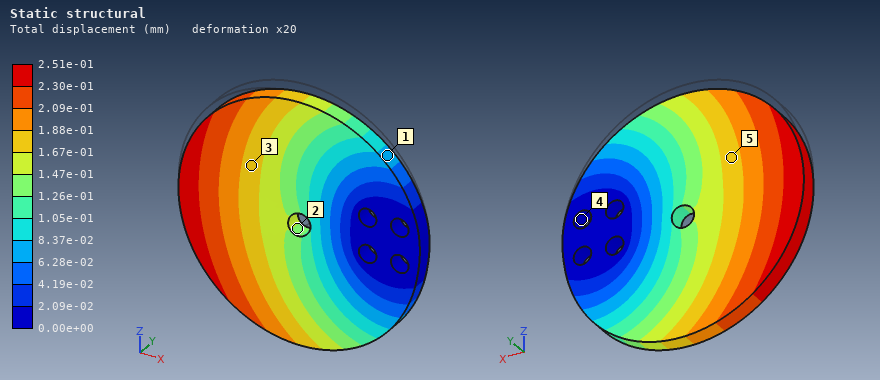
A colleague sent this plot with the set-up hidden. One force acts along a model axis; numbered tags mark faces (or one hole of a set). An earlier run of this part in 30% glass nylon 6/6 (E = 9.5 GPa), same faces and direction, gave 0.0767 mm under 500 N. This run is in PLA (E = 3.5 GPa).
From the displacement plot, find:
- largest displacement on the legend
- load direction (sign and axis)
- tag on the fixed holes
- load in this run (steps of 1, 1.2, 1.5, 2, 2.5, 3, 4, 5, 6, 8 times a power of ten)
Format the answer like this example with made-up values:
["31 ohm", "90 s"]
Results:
["2.51e-01 mm", "-Z", "4", "600 N"]
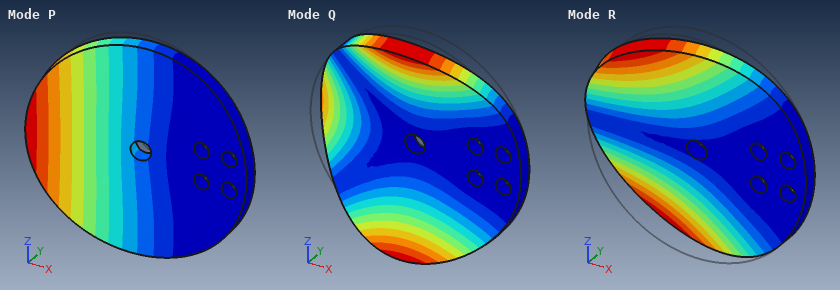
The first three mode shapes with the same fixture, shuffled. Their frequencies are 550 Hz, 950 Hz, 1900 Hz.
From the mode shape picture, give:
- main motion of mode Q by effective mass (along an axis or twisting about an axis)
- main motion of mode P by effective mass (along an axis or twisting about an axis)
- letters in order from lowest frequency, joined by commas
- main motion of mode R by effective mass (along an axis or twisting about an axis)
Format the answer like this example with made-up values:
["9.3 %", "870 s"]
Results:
["along Y", "along Y", "P, R, Q", "twisting about X"]
